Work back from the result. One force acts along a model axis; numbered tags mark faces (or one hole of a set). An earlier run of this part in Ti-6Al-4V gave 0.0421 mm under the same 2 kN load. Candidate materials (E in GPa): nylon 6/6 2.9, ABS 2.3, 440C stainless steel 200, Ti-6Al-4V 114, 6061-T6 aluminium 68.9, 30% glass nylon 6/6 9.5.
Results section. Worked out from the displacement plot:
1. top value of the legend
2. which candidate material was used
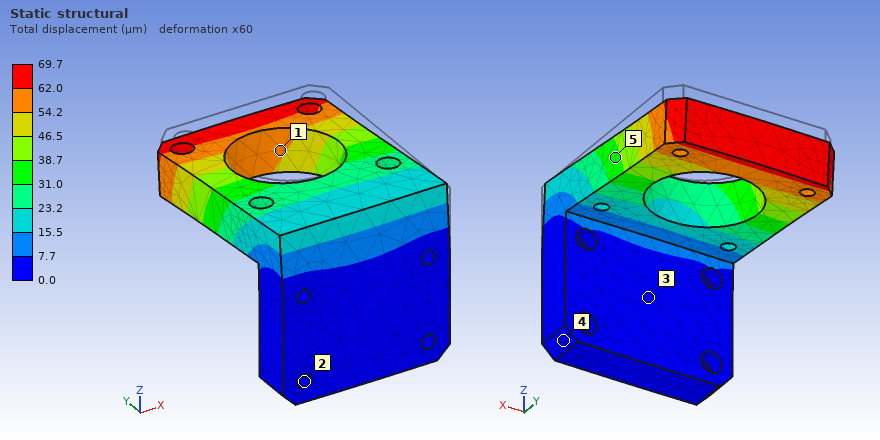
69.7 µm
6061-T6 aluminium
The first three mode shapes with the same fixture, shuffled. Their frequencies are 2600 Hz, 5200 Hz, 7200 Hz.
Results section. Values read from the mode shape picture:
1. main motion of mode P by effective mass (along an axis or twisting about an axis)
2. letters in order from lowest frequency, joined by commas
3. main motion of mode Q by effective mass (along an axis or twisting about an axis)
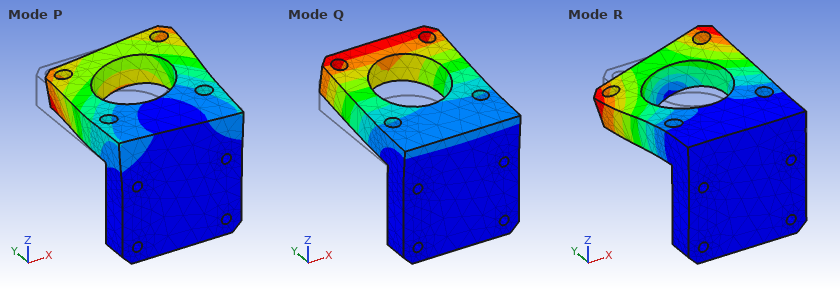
along X
Q, P, R
along Z
